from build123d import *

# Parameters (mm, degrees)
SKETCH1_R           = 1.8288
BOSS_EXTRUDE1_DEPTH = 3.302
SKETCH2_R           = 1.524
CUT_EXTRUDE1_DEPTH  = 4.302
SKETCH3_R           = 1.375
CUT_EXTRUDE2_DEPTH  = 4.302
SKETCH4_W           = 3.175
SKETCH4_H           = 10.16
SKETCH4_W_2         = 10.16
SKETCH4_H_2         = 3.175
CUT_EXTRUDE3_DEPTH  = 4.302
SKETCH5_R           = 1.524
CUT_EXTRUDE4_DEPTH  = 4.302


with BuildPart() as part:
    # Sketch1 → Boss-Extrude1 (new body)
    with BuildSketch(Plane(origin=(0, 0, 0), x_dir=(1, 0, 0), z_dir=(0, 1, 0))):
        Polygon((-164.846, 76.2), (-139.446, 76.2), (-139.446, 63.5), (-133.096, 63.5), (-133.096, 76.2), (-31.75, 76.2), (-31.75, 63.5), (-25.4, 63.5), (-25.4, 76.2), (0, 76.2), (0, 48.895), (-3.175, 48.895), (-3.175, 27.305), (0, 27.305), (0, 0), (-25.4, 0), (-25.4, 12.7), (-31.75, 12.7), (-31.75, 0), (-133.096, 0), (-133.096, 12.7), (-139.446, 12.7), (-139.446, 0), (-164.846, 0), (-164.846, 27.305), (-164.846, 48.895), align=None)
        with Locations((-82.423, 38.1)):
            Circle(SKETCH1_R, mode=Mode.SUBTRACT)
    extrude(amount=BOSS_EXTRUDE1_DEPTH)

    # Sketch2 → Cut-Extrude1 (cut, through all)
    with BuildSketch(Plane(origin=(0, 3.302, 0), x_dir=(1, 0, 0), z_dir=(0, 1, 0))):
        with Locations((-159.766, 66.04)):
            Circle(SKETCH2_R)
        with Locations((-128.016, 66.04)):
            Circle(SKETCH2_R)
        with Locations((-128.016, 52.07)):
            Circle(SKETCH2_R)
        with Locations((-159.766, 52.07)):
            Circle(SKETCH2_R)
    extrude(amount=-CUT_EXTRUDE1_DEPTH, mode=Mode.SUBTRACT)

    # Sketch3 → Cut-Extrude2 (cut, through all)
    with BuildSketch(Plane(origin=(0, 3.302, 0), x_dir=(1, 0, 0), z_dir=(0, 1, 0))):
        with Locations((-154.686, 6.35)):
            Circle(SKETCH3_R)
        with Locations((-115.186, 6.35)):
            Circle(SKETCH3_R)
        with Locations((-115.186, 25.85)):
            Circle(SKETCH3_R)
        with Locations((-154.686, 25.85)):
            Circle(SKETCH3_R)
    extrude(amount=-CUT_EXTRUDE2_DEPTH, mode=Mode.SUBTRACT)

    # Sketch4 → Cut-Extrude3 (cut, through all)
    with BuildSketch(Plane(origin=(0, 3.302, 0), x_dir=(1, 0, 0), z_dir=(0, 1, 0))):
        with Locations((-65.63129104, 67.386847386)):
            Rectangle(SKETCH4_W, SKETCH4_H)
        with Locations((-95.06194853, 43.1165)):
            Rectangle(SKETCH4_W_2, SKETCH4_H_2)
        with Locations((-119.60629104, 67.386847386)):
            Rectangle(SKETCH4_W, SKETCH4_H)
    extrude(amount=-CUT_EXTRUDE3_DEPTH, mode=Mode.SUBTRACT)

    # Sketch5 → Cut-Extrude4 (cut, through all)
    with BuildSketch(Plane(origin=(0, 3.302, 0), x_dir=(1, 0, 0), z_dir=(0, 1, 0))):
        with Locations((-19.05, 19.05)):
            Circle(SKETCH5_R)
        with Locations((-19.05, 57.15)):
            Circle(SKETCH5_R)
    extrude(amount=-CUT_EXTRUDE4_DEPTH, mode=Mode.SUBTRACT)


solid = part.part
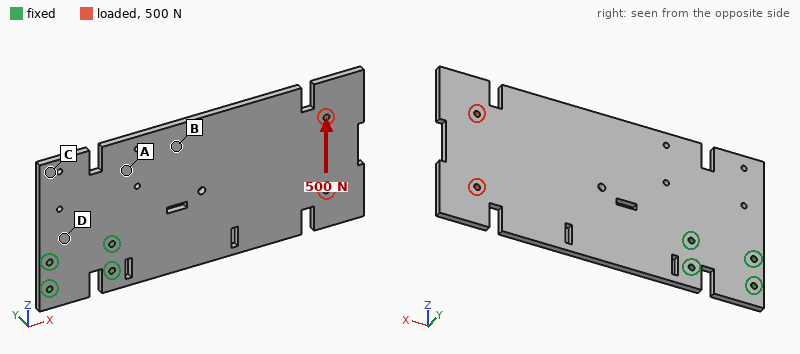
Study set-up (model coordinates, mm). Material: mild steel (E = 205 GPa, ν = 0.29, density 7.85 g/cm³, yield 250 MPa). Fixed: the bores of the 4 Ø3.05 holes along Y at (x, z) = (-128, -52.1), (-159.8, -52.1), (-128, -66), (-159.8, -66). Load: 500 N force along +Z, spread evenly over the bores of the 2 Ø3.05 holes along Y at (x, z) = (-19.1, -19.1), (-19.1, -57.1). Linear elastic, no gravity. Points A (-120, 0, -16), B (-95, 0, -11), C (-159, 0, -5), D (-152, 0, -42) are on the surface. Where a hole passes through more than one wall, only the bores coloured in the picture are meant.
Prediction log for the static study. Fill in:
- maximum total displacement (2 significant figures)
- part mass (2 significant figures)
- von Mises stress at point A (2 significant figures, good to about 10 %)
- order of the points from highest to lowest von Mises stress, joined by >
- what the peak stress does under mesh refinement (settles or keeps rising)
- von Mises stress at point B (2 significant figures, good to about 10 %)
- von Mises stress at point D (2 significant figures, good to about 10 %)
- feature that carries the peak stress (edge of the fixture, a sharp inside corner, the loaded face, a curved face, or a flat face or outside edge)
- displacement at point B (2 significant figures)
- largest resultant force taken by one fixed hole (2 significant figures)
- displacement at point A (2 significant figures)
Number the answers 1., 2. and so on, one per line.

1. 48 µm
2. 310 g
3. 15 MPa
4. D > A > B > C
5. keeps rising
6. 8.8 MPa
7. 21 MPa
8. edge of the fixture
9. 16 µm
10. 1.3 kN
11. 9.5 µm
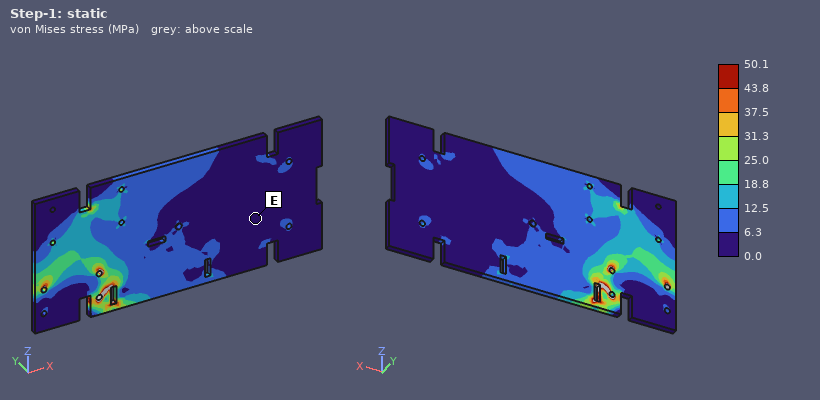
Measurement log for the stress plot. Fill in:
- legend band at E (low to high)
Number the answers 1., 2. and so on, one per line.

1. 0.0 to 6.3 MPa
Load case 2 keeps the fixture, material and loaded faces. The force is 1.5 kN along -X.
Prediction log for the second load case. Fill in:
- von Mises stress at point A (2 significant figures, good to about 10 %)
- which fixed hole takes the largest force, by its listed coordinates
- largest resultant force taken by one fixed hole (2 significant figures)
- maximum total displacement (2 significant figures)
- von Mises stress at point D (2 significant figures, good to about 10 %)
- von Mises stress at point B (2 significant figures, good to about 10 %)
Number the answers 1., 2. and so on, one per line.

1. 7.3 MPa
2. (-128, -52.1)
3. 1.1 kN
4. 16 µm
5. 13 MPa
6. 5.5 MPa
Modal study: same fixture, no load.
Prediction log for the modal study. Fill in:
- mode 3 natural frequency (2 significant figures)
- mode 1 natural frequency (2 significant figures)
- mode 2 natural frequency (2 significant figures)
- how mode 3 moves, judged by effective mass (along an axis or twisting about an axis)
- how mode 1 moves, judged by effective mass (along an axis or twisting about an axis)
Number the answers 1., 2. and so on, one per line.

1. 880 Hz
2. 150 Hz
3. 490 Hz
4. along Y
5. along Y
